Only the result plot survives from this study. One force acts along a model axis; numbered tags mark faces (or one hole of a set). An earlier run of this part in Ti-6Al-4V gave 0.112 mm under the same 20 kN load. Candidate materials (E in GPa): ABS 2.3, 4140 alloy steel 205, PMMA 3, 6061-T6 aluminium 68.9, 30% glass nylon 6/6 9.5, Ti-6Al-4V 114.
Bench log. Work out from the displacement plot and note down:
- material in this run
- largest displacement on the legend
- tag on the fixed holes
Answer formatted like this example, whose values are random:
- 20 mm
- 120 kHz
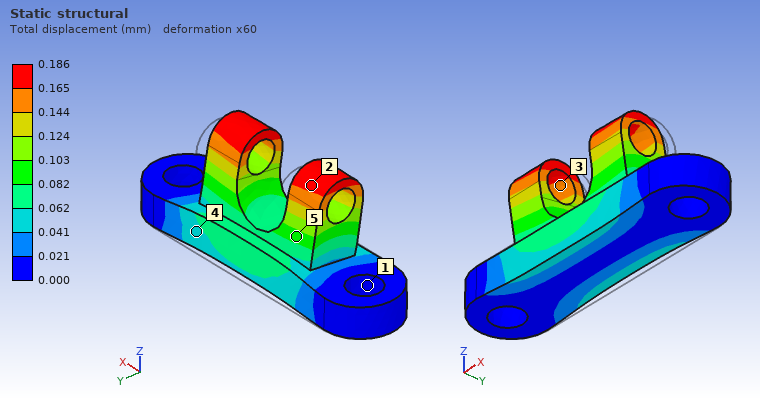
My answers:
- 6061-T6 aluminium
- 0.186 mm
- 1
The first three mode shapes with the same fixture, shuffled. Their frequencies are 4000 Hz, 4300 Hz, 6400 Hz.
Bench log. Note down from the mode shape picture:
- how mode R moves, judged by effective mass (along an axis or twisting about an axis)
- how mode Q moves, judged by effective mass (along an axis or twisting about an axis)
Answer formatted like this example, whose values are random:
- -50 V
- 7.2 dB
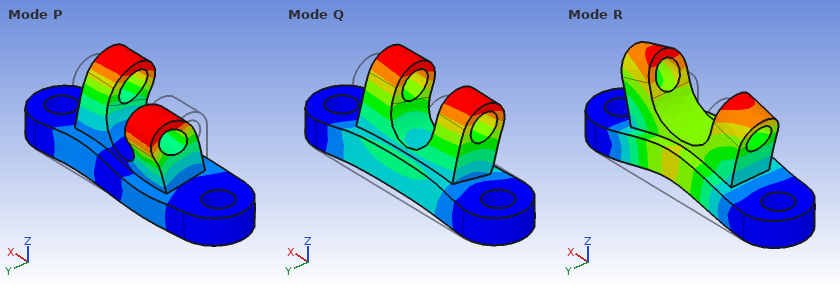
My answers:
- along Z
- along Y
